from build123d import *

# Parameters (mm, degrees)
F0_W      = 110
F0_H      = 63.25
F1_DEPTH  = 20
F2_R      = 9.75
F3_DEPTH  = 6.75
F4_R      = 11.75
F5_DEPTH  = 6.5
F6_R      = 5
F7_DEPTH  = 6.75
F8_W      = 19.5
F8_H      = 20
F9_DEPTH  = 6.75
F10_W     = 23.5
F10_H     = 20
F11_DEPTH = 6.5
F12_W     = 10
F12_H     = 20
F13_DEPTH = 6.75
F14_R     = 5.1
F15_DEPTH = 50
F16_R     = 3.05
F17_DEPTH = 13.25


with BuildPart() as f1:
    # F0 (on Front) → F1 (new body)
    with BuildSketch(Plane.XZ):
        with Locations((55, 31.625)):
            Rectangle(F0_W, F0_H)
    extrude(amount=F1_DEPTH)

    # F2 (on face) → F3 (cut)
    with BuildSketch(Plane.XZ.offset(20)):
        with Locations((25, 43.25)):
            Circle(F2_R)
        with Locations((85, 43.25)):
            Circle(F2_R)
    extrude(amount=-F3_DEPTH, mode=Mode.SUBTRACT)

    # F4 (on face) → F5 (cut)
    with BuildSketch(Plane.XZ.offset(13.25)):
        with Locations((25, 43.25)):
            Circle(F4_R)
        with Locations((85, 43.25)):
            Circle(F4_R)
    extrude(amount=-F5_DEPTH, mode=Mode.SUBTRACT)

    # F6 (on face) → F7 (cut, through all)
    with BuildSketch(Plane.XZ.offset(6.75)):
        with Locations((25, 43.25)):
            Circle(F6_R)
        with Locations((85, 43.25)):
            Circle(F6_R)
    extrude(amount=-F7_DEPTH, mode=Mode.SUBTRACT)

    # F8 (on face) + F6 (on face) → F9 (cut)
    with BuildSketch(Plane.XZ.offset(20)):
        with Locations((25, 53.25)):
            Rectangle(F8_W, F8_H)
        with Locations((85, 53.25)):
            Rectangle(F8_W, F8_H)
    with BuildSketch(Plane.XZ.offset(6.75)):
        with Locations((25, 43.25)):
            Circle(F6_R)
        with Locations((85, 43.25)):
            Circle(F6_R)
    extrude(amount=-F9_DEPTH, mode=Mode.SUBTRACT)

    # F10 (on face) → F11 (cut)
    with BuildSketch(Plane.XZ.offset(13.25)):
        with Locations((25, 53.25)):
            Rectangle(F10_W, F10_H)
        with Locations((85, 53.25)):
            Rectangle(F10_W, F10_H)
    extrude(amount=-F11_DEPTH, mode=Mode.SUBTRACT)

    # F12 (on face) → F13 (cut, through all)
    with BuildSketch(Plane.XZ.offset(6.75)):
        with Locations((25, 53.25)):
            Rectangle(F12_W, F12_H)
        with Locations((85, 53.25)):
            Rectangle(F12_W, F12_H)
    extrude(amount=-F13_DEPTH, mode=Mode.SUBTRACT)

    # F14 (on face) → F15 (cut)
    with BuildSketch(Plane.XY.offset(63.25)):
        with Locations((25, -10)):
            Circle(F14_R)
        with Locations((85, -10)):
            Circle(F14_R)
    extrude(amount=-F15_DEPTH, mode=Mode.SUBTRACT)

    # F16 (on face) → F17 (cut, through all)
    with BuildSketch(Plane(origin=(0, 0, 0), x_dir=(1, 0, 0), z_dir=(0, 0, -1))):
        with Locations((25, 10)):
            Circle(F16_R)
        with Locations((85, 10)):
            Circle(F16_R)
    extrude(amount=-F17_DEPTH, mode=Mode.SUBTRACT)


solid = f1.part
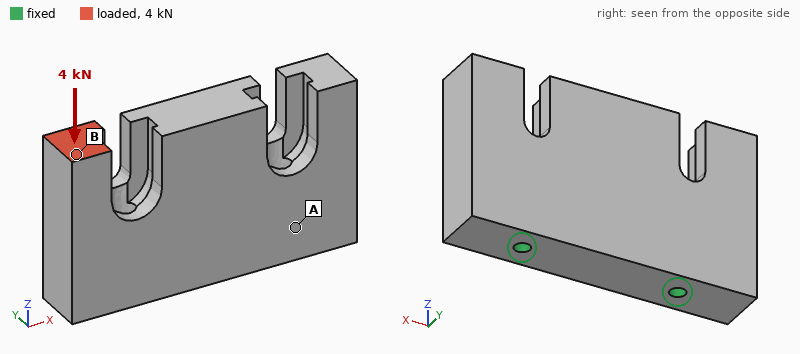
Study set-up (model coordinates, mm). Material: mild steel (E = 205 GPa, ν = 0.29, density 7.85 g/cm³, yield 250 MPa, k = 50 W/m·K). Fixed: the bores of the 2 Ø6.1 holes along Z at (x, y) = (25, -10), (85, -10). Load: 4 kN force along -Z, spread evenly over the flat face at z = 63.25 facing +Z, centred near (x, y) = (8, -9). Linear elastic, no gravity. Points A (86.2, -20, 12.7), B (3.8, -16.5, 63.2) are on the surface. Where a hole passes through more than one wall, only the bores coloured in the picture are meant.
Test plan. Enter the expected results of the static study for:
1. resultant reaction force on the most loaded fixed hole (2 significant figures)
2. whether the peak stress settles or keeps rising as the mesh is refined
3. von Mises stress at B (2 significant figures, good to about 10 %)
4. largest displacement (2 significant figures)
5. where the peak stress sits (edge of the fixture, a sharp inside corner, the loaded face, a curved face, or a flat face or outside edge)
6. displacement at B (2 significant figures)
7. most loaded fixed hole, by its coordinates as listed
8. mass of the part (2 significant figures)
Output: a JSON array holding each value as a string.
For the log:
["4.8 kN", "keeps rising", "12 MPa", "11 µm", "edge of the fixture", "10 µm", "(25, -10)", "910 g"]
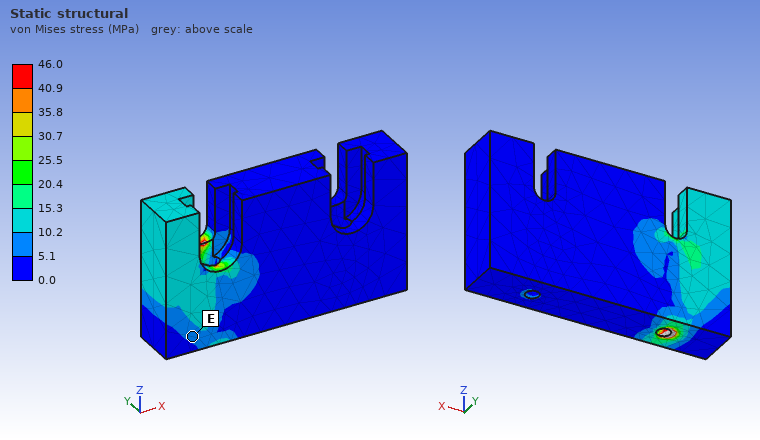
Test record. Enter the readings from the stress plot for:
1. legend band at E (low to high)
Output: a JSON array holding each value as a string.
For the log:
["5.1 to 10.2 MPa"]
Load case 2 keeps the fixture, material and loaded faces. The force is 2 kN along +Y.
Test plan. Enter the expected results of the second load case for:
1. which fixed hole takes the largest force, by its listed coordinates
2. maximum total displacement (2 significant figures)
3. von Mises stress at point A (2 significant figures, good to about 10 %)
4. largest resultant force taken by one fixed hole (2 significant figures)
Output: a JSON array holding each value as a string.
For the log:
["(25, -10)", "66 µm", "16 MPa", "2.3 kN"]
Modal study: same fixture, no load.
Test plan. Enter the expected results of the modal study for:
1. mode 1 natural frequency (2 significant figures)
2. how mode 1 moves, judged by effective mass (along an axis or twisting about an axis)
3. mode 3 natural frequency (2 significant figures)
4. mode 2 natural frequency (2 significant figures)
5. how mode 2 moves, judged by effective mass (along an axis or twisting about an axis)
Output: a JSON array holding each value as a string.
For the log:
["3000 Hz", "along Y", "5500 Hz", "4500 Hz", "twisting about Z"]
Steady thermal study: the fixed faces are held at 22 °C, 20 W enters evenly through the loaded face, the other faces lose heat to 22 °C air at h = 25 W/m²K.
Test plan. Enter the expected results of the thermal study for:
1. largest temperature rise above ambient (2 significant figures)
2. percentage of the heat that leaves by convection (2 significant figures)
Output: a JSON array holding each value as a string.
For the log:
["54 K", "20 %"]
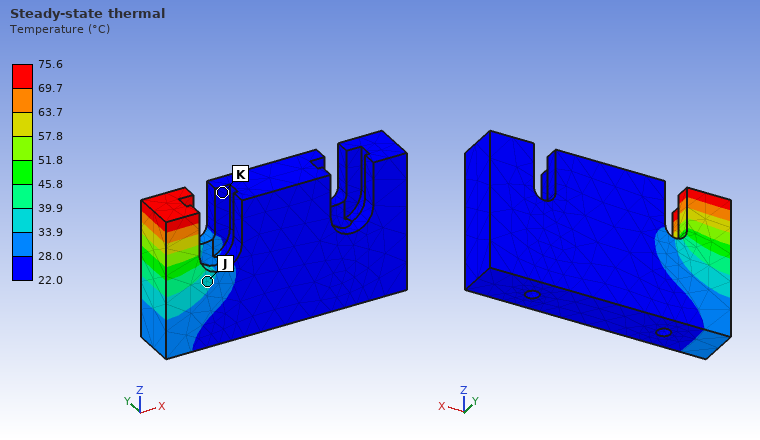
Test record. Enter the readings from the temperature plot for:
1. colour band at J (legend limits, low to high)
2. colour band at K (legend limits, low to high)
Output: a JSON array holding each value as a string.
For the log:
["33.9 to 39.9 °C", "22.0 to 28.0 °C"]
